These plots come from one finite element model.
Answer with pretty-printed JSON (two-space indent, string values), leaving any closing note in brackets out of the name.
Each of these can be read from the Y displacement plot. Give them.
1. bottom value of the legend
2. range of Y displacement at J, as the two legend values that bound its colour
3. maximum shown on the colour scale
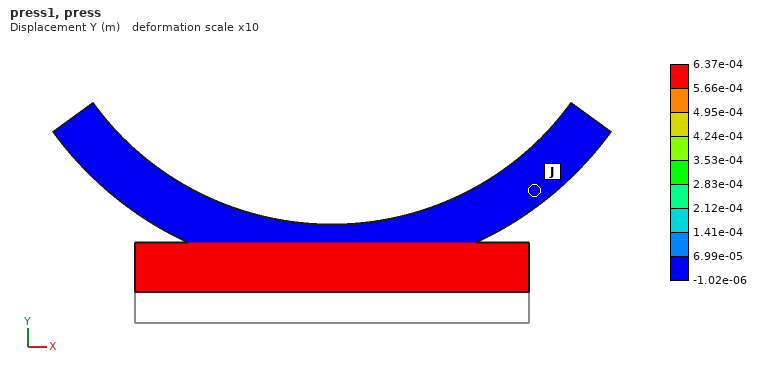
{
  "bottom value of the legend": "-1.02e-06 m",
  "range of Y displacement at J, as the two legend values that bound its colour": "-1.02e-06 to 6.99e-05 m",
  "maximum shown on the colour scale": "6.37e-04 m"
}
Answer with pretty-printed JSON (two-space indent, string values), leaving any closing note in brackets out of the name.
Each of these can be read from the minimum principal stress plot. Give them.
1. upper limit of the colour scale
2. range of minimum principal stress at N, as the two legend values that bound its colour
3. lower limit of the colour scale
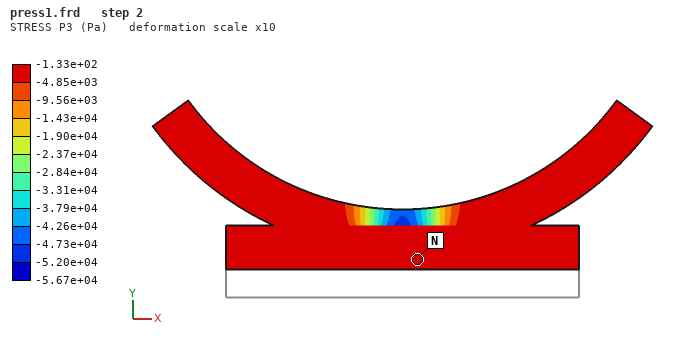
{
  "upper limit of the colour scale": "-1.33e+02 Pa",
  "range of minimum principal stress at N, as the two legend values that bound its colour": "-4.85e+03 to -1.33e+02 Pa",
  "lower limit of the colour scale": "-5.67e+04 Pa"
}
